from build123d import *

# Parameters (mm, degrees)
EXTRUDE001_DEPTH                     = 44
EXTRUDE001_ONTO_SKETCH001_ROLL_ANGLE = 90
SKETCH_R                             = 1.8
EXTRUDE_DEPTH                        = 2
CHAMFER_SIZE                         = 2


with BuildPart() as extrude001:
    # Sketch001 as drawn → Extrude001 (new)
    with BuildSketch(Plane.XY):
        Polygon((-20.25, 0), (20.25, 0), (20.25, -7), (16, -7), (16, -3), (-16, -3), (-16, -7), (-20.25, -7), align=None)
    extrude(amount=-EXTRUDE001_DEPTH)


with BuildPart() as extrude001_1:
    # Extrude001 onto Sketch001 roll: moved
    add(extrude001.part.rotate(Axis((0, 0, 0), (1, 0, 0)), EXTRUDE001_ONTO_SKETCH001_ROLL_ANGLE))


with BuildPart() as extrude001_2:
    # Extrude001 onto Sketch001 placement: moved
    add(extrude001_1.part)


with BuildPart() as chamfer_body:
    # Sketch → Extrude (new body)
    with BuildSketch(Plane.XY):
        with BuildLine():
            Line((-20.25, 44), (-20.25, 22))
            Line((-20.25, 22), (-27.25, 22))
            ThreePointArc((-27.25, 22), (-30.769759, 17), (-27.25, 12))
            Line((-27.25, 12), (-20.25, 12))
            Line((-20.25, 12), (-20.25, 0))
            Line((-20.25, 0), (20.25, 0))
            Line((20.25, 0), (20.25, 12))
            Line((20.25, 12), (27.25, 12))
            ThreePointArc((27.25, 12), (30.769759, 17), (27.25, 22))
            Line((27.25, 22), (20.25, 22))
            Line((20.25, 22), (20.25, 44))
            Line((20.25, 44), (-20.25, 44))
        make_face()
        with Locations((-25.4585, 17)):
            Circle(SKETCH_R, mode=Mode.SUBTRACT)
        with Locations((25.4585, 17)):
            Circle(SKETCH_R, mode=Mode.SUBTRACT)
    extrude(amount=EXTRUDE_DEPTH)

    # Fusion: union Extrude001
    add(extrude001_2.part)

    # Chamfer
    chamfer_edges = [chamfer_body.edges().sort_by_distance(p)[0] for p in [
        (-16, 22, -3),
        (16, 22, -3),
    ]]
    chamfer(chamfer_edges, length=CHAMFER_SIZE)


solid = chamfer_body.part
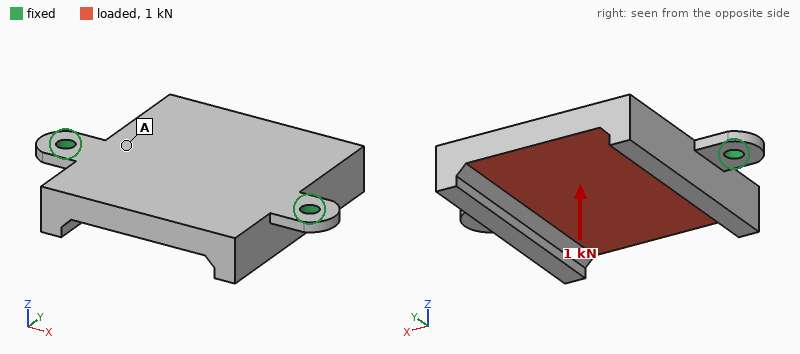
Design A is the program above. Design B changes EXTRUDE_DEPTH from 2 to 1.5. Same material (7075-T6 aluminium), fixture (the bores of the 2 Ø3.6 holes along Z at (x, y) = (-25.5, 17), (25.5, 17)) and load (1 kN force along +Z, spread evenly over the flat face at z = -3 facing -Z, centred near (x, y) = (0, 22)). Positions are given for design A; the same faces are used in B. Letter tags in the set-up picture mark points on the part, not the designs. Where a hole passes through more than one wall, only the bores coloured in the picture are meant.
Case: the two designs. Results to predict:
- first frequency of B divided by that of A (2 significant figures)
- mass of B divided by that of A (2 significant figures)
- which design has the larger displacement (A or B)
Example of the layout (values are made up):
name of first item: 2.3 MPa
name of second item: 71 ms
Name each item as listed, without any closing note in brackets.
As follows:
first frequency of B divided by that of A: 0.75
mass of B divided by that of A: 0.91
which design has the larger displacement: B
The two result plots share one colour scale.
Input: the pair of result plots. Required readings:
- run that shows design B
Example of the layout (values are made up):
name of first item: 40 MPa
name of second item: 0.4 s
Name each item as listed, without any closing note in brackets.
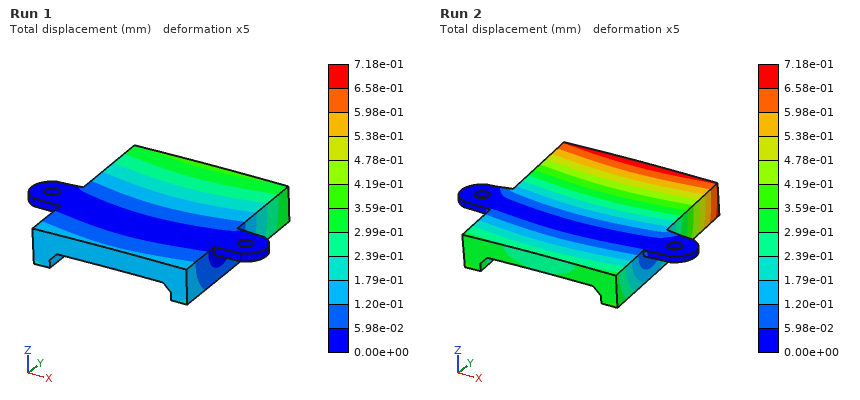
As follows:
run that shows design B: Run 2
